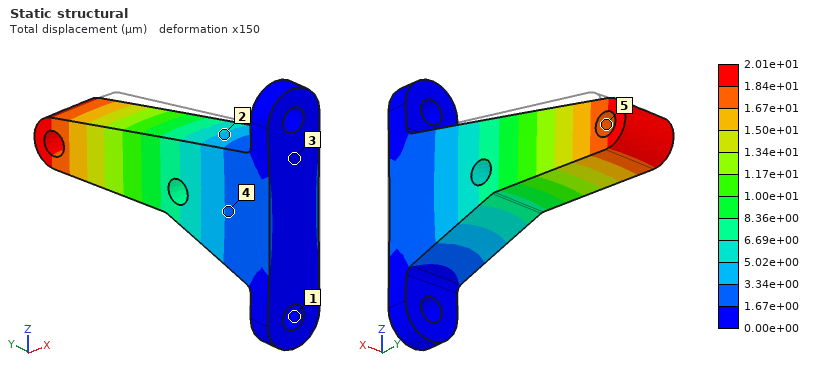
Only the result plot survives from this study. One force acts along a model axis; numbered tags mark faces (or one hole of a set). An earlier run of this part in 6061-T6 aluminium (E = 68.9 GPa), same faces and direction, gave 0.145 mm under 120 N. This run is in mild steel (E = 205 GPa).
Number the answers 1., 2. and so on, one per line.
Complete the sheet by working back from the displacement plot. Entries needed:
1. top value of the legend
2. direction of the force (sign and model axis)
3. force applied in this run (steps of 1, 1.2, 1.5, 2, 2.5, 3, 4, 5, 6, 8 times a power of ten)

1. 2.01e+01 µm
2. -X
3. 50 N
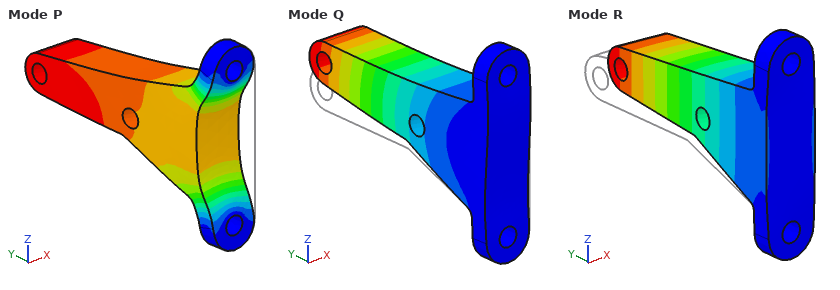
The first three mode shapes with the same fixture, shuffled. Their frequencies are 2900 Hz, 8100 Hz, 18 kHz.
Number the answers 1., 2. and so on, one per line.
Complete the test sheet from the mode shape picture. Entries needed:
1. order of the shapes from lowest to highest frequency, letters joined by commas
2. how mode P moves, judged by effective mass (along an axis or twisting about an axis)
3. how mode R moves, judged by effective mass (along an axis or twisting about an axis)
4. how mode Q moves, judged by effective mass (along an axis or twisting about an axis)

1. R, Q, P
2. along Y
3. along X
4. along Z
